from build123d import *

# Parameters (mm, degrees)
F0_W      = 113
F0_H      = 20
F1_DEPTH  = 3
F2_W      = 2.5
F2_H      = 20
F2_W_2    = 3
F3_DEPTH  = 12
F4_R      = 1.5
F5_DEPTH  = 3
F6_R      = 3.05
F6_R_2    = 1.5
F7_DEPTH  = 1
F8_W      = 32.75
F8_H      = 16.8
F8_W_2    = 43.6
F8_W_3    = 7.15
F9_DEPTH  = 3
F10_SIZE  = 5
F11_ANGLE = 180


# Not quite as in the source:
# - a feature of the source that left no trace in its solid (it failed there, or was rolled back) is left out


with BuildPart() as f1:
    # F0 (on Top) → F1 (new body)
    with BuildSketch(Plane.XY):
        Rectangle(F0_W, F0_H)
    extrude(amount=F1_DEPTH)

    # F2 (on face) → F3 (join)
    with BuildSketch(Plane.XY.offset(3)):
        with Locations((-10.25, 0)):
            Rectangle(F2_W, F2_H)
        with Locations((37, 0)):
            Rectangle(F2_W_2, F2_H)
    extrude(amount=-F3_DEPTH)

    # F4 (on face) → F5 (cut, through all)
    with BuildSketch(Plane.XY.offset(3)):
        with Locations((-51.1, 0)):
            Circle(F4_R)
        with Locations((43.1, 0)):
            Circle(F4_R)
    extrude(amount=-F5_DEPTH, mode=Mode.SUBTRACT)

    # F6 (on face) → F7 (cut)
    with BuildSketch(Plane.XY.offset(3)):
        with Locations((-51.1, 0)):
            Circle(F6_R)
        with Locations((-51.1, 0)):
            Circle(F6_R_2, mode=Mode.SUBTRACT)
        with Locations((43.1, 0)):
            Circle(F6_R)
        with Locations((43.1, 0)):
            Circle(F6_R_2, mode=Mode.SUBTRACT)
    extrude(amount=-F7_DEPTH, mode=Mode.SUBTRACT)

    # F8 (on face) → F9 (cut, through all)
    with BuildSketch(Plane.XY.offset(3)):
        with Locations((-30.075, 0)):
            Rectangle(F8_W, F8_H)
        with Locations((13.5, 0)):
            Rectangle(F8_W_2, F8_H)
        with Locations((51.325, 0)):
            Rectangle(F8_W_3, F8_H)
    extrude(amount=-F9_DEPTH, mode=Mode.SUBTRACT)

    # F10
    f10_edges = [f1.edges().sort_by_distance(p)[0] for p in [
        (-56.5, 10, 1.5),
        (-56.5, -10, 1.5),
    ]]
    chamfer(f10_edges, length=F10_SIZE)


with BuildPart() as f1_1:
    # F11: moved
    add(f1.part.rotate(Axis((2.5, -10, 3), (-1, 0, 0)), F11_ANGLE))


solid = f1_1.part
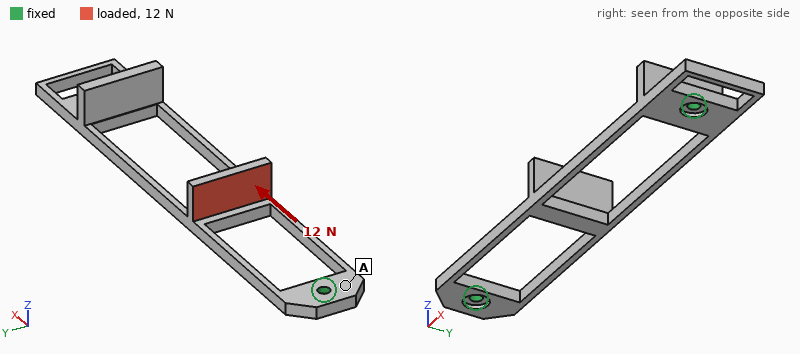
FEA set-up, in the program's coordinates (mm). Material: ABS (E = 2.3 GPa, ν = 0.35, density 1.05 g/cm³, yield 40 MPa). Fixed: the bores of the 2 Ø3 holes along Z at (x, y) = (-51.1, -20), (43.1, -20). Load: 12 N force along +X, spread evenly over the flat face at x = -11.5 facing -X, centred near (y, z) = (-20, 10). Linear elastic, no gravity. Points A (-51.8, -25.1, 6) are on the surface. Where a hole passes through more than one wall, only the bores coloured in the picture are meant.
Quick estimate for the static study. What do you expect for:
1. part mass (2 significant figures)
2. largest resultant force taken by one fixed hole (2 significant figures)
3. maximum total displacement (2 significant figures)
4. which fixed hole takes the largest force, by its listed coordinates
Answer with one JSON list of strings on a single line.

["3.6 g", "6.6 N", "0.33 mm", "(-51.1, -20)"]
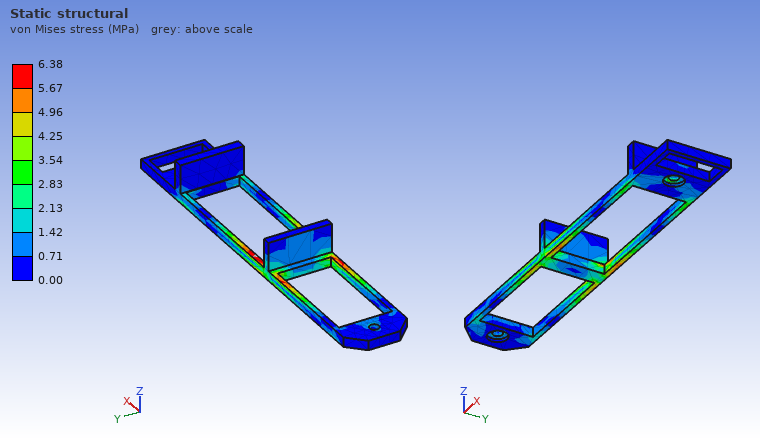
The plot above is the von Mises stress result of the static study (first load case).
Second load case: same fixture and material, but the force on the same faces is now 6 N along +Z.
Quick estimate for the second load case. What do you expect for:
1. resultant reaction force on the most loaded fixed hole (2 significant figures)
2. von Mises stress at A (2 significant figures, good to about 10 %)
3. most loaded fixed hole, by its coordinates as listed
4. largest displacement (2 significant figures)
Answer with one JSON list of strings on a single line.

["3.6 N", "2.5 MPa", "(-51.1, -20)", "1.2 mm"]
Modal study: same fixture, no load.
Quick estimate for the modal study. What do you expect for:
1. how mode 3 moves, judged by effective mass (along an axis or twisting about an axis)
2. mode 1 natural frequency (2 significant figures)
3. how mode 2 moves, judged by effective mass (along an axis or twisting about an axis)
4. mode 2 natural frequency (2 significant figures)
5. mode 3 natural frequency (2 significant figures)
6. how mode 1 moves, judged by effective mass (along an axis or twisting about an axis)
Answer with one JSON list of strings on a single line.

["twisting about X", "210 Hz", "along Z", "340 Hz", "520 Hz", "along Y"]
